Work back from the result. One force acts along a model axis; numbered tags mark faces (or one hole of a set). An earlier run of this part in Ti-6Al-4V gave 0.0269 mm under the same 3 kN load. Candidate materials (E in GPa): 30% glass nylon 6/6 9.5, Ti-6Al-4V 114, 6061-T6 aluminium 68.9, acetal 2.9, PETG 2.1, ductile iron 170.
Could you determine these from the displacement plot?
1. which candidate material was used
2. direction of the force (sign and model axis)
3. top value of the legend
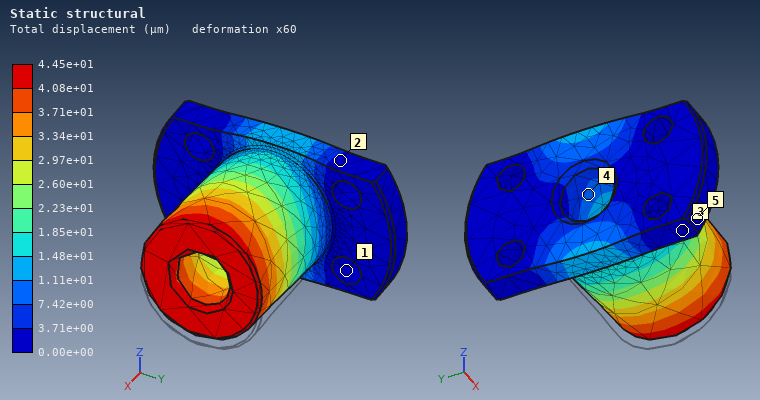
6061-T6 aluminium
+Z
4.45e+01 µm
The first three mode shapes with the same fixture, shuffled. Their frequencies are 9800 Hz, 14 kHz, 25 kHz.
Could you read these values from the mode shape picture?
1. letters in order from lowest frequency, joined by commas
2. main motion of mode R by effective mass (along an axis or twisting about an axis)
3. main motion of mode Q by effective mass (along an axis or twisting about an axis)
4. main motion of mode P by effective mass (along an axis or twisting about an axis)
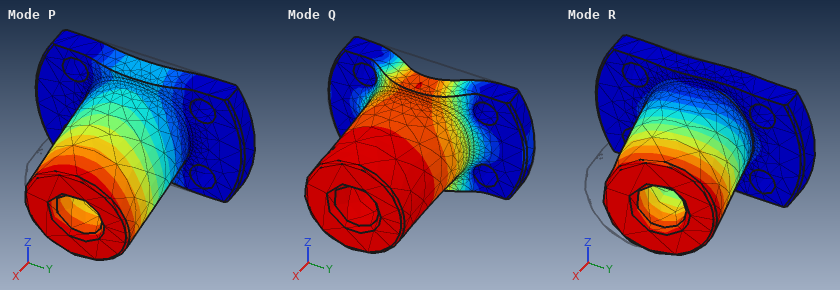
P, R, Q
along Y
along X
along Z
